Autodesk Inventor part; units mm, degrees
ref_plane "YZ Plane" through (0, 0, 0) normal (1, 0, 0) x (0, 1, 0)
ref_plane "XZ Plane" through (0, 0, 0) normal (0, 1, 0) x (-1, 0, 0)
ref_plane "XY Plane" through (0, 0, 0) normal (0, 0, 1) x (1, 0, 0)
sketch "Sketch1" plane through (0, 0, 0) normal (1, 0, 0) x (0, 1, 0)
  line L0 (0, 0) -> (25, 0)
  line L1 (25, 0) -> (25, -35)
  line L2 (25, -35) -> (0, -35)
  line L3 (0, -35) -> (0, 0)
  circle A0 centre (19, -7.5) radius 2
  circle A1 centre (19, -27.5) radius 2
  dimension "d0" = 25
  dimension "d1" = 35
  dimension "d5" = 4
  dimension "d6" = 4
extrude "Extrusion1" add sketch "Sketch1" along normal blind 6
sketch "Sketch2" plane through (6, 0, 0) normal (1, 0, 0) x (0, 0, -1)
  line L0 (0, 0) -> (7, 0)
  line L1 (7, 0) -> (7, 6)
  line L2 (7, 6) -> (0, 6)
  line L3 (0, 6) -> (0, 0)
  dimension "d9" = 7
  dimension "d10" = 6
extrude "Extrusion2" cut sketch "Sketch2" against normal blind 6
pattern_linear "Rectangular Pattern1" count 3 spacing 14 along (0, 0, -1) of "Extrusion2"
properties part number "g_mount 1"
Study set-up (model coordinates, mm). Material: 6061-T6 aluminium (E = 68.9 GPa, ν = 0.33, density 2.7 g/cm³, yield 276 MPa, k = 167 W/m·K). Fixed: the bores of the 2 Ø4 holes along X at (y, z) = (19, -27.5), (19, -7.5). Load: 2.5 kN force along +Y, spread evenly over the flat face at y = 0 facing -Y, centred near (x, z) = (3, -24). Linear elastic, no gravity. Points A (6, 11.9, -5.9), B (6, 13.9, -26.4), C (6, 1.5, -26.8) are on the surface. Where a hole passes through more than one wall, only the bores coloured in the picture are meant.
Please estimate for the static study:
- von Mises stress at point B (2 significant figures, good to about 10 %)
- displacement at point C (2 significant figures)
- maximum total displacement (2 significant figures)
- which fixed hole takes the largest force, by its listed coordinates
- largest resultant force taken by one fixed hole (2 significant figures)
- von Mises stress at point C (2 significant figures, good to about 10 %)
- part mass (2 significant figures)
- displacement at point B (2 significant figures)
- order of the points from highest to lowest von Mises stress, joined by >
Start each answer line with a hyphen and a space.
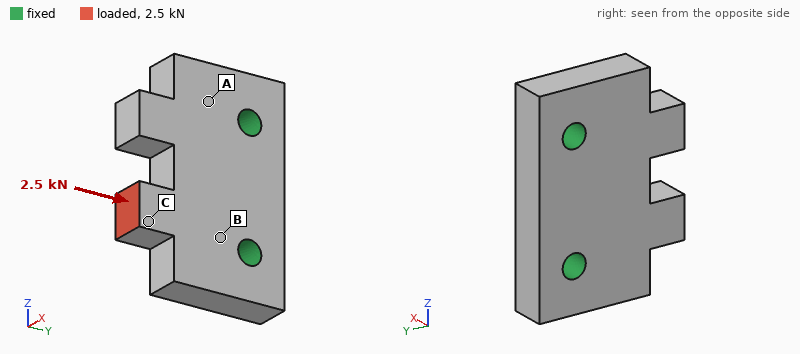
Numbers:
- 45 MPa
- 11 µm
- 12 µm
- (19, -27.5)
- 2.1 kN
- 58 MPa
- 12 g
- 2.3 µm
- C > B > A
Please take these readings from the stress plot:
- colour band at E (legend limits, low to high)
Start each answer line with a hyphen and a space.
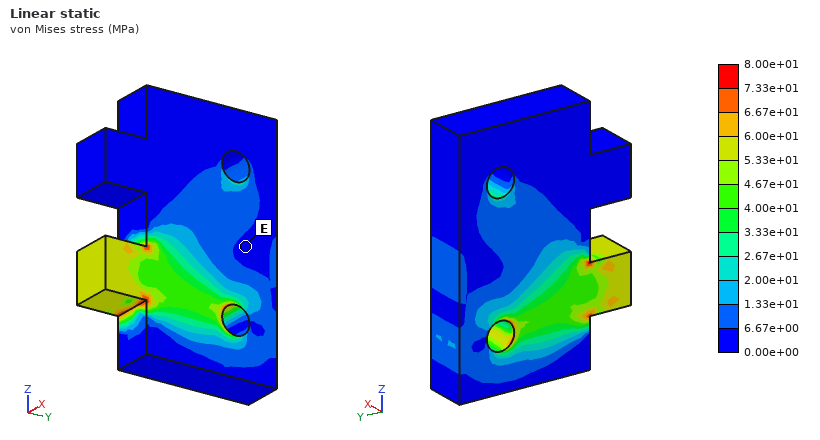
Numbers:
- 0.00e+00 to 6.67e+00 MPa
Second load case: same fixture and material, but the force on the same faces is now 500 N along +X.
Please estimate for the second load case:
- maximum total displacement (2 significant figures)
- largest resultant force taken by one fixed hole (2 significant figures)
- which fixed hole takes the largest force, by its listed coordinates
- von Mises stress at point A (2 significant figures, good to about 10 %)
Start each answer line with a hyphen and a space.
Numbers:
- 60 µm
- 420 N
- (19, -27.5)
- 17 MPa
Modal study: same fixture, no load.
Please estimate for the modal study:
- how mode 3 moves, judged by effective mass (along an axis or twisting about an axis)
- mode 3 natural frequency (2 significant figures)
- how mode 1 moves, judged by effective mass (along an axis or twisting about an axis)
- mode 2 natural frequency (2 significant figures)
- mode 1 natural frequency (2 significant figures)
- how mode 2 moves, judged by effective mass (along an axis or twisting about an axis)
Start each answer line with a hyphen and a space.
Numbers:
- along Z
- 36 kHz
- along X
- 23 kHz
- 16 kHz
- twisting about Y
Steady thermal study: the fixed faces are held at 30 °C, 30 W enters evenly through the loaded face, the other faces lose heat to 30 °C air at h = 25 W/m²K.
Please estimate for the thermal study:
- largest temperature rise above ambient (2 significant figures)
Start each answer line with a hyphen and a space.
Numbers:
- 50 K
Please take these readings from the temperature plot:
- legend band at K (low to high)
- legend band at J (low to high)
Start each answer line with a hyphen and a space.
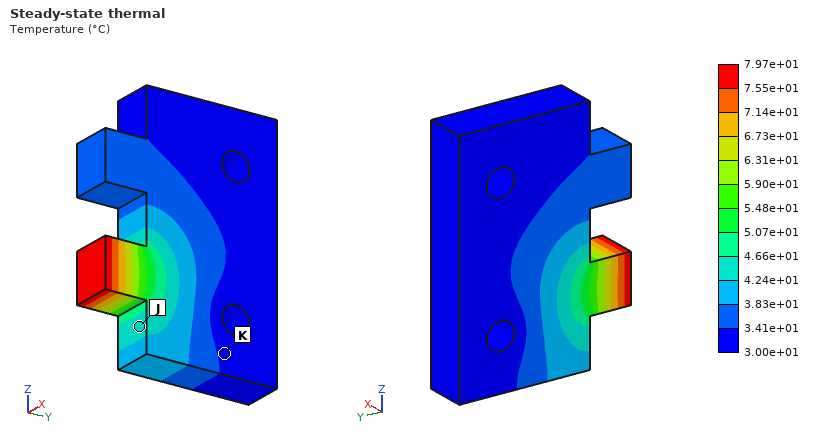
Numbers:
- 3.00e+01 to 3.41e+01 °C
- 4.24e+01 to 4.66e+01 °C
